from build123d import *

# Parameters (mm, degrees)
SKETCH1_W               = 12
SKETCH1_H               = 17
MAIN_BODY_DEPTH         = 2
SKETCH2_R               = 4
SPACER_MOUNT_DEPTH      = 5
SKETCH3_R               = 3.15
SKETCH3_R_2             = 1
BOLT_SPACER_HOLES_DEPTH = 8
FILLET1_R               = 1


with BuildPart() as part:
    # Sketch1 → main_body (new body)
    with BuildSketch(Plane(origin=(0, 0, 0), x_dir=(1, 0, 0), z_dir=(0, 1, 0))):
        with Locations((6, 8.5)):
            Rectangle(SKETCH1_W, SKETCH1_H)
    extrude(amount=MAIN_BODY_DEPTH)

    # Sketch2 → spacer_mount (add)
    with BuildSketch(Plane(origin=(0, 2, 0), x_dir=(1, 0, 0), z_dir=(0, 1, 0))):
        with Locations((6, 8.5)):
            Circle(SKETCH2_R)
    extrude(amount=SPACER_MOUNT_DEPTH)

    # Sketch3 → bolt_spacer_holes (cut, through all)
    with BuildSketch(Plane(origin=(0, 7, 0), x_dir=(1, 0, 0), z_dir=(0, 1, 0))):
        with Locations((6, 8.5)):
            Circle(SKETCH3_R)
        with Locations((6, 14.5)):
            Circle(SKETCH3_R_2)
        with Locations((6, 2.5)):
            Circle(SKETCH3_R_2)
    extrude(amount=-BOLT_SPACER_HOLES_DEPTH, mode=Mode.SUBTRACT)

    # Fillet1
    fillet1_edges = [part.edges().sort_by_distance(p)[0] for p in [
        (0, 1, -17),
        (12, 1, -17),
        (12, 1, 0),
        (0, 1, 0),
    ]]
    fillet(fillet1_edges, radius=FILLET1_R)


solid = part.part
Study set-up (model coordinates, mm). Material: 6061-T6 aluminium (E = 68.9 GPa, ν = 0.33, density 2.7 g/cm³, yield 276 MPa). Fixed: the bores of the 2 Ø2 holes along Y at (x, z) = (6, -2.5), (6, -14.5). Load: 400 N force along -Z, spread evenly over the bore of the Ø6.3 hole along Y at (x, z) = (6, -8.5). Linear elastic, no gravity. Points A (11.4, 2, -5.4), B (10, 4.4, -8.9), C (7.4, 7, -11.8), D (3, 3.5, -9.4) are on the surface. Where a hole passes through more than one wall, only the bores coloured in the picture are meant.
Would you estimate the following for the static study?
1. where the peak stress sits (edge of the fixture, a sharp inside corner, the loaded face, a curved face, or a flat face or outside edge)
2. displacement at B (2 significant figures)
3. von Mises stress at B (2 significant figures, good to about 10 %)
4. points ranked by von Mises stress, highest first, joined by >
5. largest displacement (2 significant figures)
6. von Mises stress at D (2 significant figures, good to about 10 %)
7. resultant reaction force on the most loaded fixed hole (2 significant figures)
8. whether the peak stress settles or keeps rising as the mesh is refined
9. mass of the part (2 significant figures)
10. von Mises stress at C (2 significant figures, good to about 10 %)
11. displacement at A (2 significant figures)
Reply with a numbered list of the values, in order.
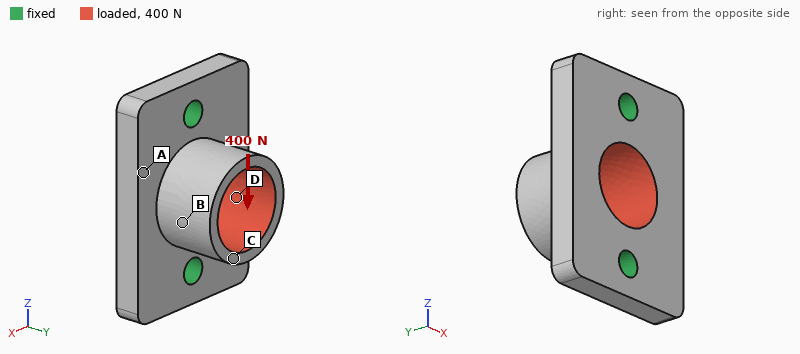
1. edge of the fixture
2. 4.1 µm
3. 23 MPa
4. D > B > C > A
5. 7.0 µm
6. 37 MPa
7. 230 N
8. keeps rising
9. 1.2 g
10. 16 MPa
11. 1.6 µm
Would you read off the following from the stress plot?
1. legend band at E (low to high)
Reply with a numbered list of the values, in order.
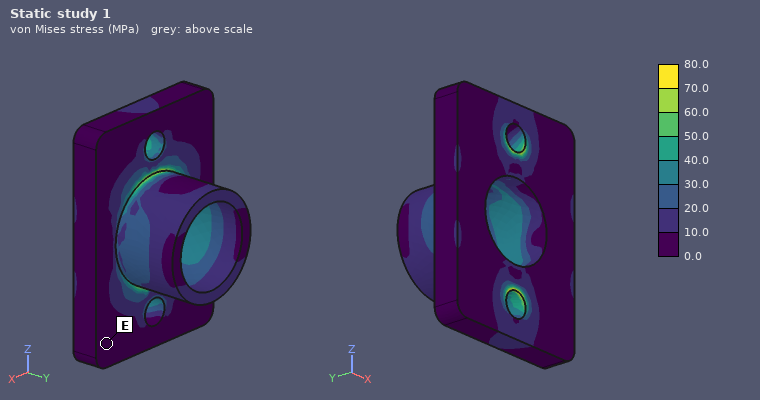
1. 0.0 to 10.0 MPa
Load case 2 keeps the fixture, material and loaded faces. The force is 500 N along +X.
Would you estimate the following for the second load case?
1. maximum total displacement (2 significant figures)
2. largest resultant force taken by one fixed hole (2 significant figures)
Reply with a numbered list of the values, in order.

1. 28 µm
2. 250 N
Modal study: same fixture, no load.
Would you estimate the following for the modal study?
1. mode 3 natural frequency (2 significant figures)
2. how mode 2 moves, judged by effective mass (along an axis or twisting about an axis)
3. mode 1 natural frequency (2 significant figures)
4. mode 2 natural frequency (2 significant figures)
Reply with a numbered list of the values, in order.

1. 54 kHz
2. along Y
3. 29 kHz
4. 41 kHz
